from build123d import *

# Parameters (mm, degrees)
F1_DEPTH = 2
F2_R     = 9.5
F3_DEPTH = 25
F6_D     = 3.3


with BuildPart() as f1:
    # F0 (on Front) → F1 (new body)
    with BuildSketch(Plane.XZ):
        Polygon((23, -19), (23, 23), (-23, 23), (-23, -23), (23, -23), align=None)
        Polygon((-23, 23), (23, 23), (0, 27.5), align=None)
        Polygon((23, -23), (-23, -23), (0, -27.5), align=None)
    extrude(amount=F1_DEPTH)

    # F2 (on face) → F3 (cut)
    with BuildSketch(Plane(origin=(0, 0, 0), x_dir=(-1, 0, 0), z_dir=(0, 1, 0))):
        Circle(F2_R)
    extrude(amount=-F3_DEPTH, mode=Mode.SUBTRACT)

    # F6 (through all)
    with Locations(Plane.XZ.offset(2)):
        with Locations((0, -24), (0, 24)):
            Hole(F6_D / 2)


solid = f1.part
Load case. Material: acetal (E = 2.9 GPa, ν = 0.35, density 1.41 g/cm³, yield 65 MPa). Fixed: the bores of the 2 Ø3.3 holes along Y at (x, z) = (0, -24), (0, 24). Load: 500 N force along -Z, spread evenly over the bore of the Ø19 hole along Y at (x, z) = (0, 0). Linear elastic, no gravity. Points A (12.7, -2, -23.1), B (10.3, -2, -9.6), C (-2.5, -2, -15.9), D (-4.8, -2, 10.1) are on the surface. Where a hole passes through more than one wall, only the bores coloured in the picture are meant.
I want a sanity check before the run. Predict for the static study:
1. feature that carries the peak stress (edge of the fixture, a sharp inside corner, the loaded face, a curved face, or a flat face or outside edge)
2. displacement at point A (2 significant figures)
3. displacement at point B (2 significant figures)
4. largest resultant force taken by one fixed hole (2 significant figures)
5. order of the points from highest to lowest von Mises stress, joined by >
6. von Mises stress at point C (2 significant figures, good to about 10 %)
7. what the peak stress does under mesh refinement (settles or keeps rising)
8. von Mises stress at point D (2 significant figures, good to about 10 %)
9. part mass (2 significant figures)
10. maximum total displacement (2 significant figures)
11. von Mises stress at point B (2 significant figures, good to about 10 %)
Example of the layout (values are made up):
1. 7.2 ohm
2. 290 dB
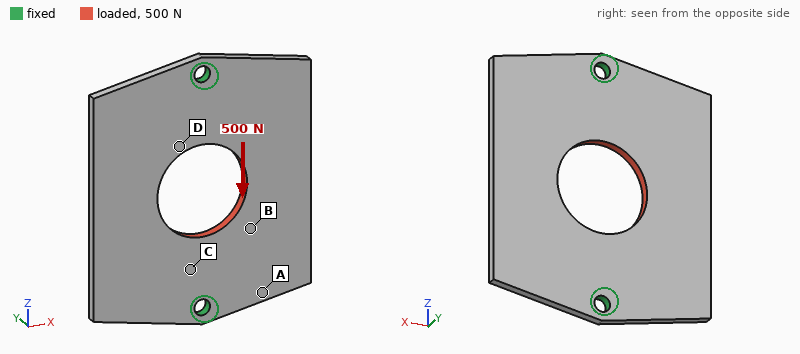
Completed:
1. edge of the fixture
2. 47 µm
3. 55 µm
4. 250 N
5. C > D > B > A
6. 8.4 MPa
7. keeps rising
8. 6.9 MPa
9. 5.7 g
10. 69 µm
11. 4.1 MPa
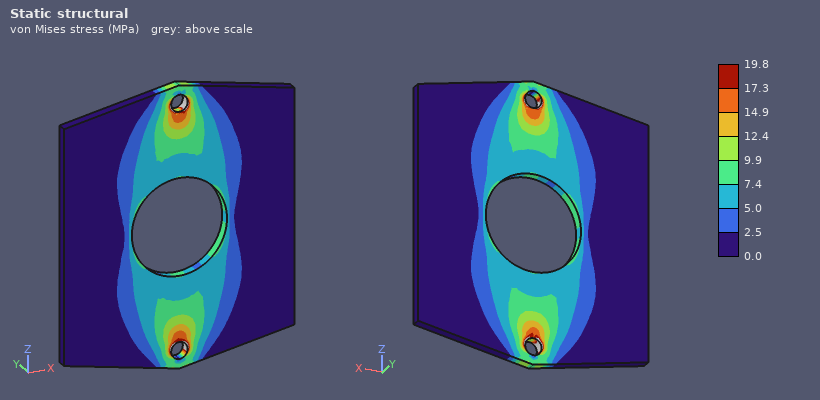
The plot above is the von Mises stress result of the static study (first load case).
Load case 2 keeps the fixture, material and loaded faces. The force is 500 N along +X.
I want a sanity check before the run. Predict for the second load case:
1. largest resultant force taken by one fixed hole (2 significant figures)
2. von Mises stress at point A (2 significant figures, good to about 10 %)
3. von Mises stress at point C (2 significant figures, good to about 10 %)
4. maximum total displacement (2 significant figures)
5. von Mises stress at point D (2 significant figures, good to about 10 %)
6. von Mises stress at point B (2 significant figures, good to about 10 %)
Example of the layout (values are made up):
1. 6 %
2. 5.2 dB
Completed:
1. 250 N
2. 3.6 MPa
3. 6.4 MPa
4. 97 µm
5. 6.8 MPa
6. 5.7 MPa
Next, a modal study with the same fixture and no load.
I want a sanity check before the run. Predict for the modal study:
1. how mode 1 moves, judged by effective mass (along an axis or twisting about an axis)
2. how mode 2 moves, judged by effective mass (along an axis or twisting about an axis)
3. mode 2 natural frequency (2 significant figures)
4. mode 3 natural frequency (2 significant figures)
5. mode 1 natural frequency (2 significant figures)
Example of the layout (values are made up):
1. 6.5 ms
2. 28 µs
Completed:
1. twisting about Z
2. along Y
3. 700 Hz
4. 1300 Hz
5. 540 Hz
